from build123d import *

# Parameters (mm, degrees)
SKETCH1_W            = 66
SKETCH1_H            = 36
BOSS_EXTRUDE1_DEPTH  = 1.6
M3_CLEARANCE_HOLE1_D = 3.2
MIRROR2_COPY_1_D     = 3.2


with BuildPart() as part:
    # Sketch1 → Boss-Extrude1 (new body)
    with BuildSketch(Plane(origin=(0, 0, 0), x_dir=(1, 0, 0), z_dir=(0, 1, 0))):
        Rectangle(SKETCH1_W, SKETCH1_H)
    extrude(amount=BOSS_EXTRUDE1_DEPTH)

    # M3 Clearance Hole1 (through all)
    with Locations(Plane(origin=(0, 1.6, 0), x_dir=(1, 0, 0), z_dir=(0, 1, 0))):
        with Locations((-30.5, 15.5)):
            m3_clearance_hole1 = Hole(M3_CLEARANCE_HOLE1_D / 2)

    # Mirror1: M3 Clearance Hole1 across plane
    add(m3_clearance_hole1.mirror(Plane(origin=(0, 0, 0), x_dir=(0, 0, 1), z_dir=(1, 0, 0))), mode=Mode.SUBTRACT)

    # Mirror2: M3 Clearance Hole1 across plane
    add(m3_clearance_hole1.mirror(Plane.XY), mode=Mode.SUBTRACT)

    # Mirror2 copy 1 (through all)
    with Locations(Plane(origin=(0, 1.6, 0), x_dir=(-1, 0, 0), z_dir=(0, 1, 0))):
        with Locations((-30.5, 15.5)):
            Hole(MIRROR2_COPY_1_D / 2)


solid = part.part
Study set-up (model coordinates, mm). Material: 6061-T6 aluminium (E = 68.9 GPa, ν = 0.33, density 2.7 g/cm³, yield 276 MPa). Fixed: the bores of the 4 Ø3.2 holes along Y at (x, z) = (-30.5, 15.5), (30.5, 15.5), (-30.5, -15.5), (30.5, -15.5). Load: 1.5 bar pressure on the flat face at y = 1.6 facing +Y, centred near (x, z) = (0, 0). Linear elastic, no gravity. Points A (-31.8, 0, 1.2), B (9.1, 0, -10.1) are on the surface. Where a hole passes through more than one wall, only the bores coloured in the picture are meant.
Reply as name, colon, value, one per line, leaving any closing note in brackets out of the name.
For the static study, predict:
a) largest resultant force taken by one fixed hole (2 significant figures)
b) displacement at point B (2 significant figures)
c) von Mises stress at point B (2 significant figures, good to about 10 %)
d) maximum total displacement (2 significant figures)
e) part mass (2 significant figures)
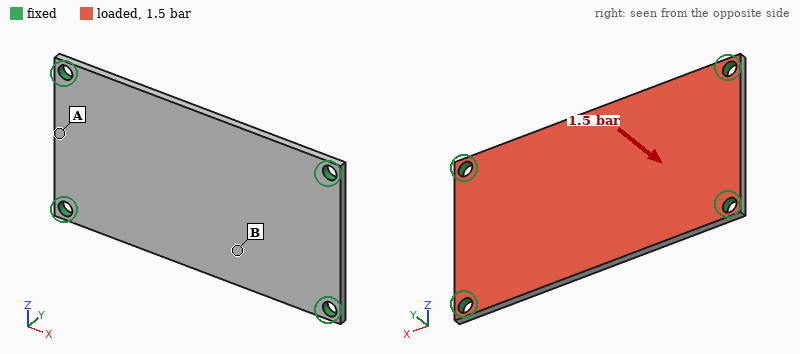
largest resultant force taken by one fixed hole: 88 N
displacement at point B: 0.23 mm
von Mises stress at point B: 44 MPa
maximum total displacement: 0.28 mm
part mass: 10 g
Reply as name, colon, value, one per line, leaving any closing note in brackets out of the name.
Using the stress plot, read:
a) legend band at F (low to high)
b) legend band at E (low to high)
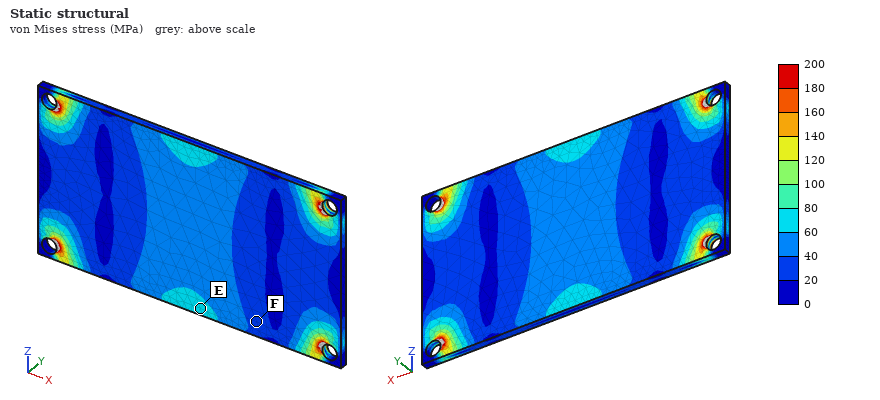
legend band at F: 20 to 40 MPa
legend band at E: 60 to 80 MPa
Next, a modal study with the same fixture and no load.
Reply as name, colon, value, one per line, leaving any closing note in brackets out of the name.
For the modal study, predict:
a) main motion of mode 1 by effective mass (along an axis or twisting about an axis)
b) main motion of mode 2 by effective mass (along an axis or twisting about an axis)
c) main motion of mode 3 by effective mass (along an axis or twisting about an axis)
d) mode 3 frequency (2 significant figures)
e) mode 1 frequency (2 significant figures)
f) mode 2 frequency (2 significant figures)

main motion of mode 1 by effective mass: along Y
main motion of mode 2 by effective mass: twisting about X
main motion of mode 3 by effective mass: twisting about Z
mode 3 frequency: 5500 Hz
mode 1 frequency: 2000 Hz
mode 2 frequency: 3500 Hz
